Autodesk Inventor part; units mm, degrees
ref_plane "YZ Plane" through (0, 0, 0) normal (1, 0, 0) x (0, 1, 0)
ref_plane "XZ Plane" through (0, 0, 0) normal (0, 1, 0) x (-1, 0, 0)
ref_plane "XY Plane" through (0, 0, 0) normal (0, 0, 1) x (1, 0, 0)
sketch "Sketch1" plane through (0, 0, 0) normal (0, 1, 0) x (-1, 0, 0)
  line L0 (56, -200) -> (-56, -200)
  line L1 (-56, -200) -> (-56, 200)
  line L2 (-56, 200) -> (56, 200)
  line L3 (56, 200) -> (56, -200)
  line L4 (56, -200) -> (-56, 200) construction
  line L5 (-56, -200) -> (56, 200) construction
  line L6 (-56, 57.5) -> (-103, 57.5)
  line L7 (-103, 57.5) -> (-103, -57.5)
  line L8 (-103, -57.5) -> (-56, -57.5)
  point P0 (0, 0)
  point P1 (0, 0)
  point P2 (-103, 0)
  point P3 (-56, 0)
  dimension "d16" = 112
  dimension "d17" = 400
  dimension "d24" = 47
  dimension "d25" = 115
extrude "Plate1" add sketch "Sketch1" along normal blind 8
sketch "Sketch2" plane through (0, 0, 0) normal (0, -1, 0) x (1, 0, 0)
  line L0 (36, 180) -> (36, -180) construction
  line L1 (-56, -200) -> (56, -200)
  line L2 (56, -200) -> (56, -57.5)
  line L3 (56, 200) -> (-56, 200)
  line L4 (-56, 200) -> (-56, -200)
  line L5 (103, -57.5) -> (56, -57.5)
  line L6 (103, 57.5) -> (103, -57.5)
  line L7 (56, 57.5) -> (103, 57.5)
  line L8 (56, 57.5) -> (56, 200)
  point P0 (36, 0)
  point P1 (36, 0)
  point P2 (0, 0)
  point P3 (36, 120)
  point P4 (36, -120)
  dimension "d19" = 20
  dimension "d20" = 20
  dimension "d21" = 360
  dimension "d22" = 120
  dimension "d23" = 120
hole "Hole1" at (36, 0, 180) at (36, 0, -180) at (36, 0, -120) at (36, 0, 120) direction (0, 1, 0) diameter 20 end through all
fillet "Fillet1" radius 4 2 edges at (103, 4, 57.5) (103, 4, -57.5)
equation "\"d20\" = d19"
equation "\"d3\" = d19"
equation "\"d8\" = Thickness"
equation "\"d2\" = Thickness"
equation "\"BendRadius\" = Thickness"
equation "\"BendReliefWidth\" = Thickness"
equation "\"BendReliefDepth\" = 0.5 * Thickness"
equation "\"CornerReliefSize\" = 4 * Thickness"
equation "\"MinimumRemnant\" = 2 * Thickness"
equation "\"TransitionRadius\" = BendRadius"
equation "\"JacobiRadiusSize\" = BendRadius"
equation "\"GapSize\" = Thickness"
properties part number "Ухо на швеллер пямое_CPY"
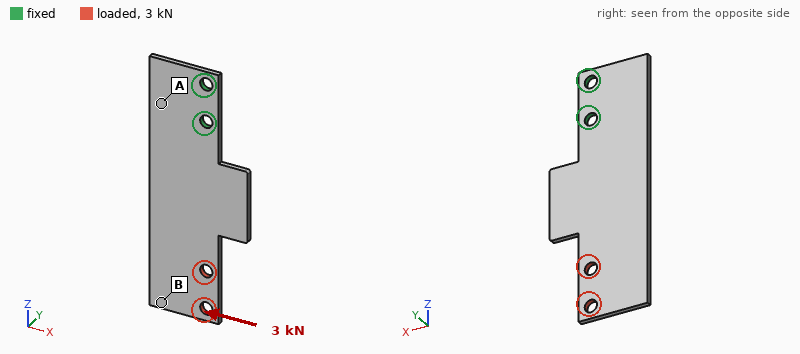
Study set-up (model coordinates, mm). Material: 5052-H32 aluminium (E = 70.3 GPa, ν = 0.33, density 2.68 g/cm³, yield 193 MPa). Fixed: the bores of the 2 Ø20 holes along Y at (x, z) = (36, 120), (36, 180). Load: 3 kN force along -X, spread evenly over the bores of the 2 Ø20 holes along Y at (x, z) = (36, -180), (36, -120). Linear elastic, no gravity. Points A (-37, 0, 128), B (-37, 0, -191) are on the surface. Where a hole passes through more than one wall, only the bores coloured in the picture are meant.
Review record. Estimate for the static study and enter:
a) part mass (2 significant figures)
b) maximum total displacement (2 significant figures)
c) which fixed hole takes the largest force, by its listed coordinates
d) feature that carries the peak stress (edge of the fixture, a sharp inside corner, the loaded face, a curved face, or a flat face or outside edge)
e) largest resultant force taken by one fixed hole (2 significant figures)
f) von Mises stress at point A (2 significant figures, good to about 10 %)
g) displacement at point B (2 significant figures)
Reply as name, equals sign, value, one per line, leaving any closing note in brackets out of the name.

part mass = 1.0 kg
maximum total displacement = 0.67 mm
which fixed hole takes the largest force, by its listed coordinates = (36, 120)
feature that carries the peak stress = edge of the fixture
largest resultant force taken by one fixed hole = 13 kN
von Mises stress at point A = 25 MPa
displacement at point B = 0.64 mm
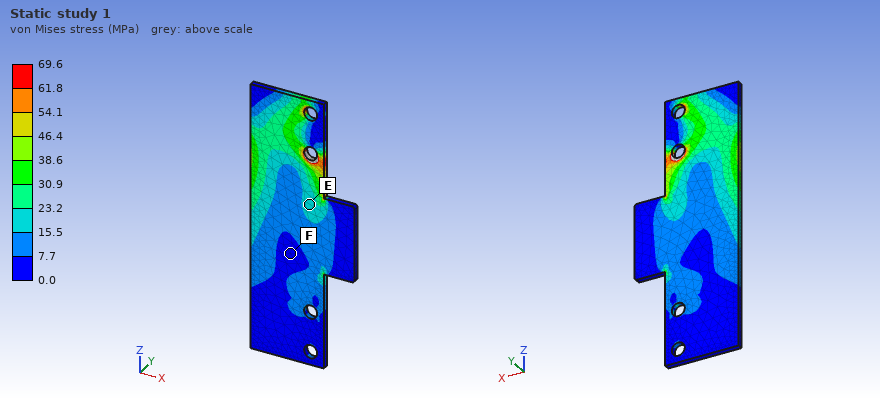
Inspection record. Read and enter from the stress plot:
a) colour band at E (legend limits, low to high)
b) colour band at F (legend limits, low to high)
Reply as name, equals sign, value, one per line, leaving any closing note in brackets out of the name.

colour band at E = 15.5 to 23.2 MPa
colour band at F = 0.0 to 7.7 MPa
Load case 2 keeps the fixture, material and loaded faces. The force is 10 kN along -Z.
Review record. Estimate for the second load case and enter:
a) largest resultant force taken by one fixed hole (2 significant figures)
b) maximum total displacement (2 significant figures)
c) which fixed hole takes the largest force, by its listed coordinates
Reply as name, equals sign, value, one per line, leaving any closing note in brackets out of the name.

largest resultant force taken by one fixed hole = 9.3 kN
maximum total displacement = 0.25 mm
which fixed hole takes the largest force, by its listed coordinates = (36, 120)
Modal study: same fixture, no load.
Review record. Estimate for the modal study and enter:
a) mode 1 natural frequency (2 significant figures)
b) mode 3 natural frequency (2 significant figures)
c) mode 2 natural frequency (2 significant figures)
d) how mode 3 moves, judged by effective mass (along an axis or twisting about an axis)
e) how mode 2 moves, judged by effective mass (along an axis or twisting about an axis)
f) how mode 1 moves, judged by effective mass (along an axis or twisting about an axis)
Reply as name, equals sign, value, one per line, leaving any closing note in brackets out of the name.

mode 1 natural frequency = 66 Hz
mode 3 natural frequency = 380 Hz
mode 2 natural frequency = 280 Hz
how mode 3 moves, judged by effective mass = along Y
how mode 2 moves, judged by effective mass = twisting about Z
how mode 1 moves, judged by effective mass = along Y
